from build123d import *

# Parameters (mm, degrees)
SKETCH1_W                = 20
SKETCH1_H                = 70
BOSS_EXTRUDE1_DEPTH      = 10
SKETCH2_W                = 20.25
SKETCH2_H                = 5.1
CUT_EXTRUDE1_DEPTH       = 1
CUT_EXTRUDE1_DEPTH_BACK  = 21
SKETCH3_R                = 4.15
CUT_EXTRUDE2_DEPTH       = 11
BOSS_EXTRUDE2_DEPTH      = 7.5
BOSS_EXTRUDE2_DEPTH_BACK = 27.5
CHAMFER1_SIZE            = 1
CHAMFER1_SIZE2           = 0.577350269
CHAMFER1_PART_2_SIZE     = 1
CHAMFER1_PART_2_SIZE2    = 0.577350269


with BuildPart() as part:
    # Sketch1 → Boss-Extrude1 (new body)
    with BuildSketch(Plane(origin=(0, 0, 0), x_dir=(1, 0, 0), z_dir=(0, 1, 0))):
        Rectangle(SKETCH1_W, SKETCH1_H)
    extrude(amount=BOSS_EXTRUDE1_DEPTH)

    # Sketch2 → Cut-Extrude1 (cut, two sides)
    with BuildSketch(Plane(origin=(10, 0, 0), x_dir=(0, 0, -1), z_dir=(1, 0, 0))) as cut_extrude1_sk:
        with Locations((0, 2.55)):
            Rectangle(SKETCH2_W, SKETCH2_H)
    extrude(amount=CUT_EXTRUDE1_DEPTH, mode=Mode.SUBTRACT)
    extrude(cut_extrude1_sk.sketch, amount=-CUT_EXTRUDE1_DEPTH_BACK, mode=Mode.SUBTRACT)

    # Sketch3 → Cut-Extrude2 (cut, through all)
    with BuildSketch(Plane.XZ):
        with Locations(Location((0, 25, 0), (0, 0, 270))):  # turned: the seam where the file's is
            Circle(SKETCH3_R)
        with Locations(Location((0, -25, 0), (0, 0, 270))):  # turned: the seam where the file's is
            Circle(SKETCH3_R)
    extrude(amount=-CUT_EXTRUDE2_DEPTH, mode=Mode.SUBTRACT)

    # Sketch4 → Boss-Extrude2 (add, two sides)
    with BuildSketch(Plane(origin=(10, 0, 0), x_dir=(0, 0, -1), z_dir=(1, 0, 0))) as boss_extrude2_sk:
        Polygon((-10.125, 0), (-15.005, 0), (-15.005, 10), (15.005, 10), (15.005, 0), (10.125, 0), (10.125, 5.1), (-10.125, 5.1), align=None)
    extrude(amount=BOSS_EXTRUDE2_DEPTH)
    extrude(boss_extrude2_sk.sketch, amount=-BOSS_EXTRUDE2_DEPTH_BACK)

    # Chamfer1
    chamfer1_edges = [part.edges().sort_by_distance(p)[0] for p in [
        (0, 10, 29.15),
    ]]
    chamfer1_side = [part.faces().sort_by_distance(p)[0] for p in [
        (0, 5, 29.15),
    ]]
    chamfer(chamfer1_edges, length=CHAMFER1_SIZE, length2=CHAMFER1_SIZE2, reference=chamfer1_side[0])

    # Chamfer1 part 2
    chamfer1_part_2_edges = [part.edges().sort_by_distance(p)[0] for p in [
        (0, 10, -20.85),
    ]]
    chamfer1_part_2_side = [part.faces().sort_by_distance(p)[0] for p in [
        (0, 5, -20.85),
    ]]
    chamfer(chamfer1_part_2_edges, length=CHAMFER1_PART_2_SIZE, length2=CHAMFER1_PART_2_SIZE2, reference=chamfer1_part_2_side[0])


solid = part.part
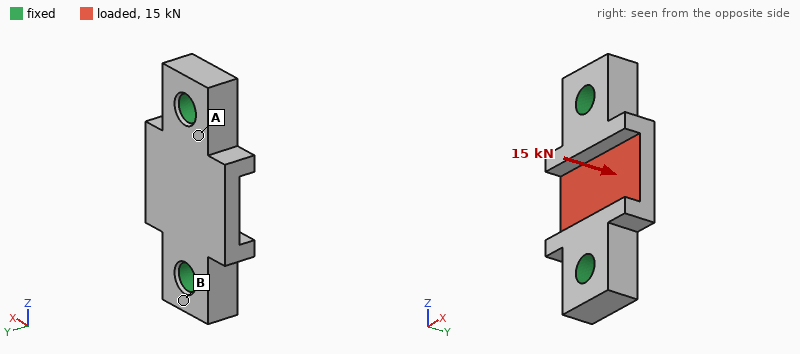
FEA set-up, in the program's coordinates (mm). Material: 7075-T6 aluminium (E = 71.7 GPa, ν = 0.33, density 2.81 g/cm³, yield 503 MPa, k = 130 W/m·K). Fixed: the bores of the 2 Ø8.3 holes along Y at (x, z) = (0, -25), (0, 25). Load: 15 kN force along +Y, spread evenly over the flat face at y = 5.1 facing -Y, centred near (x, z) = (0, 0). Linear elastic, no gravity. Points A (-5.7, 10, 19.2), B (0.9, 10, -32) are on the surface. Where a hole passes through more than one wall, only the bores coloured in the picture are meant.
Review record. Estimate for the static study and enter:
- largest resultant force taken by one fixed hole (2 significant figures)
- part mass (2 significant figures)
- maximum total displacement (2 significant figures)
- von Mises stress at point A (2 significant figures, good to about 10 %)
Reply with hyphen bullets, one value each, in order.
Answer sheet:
- 9.6 kN
- 39 g
- 0.15 mm
- 120 MPa
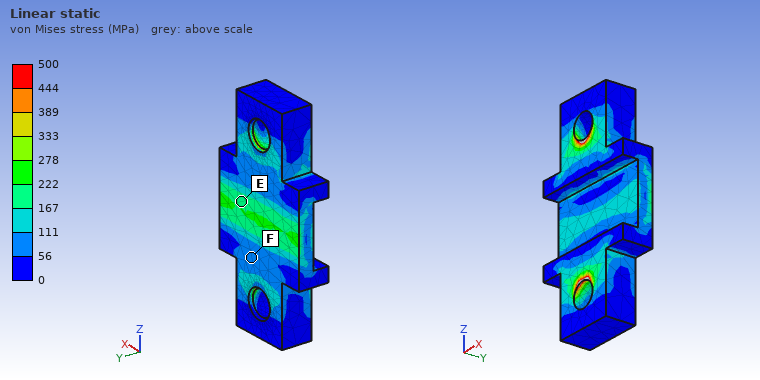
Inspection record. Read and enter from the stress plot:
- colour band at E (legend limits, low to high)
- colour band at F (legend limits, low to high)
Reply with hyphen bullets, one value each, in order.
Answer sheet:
- 167 to 222 MPa
- 56 to 111 MPa
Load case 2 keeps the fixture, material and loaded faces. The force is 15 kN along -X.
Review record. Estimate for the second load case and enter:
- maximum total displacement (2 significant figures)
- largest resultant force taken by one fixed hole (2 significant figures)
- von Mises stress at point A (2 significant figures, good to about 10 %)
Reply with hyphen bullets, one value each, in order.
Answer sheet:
- 47 µm
- 7.5 kN
- 70 MPa
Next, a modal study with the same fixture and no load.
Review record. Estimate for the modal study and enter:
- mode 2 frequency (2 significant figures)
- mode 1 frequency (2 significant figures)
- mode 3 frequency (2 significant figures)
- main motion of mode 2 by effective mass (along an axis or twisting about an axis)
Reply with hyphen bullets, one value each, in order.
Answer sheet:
- 16 kHz
- 15 kHz
- 24 kHz
- along Y
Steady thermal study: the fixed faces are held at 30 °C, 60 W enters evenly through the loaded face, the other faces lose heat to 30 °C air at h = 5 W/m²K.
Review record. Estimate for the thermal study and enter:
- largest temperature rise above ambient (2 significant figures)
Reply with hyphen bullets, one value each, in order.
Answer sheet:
- 25 K
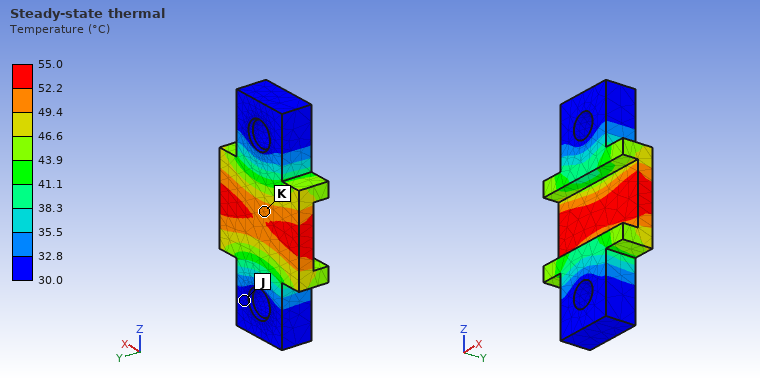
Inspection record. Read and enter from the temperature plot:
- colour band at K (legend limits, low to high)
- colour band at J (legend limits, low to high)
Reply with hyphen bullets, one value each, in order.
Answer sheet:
- 49.4 to 52.2 °C
- 30.0 to 32.8 °C
